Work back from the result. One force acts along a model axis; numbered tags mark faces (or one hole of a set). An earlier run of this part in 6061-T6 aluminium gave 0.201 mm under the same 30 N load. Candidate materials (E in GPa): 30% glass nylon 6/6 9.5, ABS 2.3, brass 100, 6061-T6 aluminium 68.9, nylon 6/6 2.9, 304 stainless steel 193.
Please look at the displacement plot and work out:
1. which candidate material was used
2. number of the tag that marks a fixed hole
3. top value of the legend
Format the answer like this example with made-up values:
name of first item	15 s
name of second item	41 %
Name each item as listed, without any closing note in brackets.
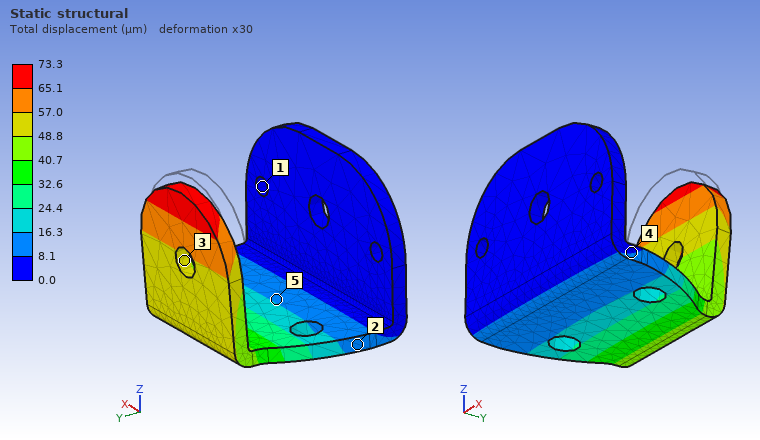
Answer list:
which candidate material was used	304 stainless steel
number of the tag that marks a fixed hole	1
top value of the legend	73.3 µm
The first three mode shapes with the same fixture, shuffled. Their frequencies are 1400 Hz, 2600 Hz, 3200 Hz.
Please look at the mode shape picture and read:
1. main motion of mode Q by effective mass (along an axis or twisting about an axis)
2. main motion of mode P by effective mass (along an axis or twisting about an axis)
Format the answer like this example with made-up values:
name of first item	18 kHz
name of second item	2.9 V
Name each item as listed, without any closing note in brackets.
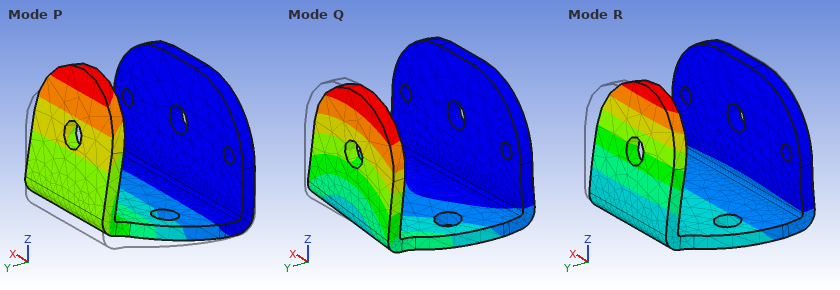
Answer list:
main motion of mode Q by effective mass	along X
main motion of mode P by effective mass	along Z
